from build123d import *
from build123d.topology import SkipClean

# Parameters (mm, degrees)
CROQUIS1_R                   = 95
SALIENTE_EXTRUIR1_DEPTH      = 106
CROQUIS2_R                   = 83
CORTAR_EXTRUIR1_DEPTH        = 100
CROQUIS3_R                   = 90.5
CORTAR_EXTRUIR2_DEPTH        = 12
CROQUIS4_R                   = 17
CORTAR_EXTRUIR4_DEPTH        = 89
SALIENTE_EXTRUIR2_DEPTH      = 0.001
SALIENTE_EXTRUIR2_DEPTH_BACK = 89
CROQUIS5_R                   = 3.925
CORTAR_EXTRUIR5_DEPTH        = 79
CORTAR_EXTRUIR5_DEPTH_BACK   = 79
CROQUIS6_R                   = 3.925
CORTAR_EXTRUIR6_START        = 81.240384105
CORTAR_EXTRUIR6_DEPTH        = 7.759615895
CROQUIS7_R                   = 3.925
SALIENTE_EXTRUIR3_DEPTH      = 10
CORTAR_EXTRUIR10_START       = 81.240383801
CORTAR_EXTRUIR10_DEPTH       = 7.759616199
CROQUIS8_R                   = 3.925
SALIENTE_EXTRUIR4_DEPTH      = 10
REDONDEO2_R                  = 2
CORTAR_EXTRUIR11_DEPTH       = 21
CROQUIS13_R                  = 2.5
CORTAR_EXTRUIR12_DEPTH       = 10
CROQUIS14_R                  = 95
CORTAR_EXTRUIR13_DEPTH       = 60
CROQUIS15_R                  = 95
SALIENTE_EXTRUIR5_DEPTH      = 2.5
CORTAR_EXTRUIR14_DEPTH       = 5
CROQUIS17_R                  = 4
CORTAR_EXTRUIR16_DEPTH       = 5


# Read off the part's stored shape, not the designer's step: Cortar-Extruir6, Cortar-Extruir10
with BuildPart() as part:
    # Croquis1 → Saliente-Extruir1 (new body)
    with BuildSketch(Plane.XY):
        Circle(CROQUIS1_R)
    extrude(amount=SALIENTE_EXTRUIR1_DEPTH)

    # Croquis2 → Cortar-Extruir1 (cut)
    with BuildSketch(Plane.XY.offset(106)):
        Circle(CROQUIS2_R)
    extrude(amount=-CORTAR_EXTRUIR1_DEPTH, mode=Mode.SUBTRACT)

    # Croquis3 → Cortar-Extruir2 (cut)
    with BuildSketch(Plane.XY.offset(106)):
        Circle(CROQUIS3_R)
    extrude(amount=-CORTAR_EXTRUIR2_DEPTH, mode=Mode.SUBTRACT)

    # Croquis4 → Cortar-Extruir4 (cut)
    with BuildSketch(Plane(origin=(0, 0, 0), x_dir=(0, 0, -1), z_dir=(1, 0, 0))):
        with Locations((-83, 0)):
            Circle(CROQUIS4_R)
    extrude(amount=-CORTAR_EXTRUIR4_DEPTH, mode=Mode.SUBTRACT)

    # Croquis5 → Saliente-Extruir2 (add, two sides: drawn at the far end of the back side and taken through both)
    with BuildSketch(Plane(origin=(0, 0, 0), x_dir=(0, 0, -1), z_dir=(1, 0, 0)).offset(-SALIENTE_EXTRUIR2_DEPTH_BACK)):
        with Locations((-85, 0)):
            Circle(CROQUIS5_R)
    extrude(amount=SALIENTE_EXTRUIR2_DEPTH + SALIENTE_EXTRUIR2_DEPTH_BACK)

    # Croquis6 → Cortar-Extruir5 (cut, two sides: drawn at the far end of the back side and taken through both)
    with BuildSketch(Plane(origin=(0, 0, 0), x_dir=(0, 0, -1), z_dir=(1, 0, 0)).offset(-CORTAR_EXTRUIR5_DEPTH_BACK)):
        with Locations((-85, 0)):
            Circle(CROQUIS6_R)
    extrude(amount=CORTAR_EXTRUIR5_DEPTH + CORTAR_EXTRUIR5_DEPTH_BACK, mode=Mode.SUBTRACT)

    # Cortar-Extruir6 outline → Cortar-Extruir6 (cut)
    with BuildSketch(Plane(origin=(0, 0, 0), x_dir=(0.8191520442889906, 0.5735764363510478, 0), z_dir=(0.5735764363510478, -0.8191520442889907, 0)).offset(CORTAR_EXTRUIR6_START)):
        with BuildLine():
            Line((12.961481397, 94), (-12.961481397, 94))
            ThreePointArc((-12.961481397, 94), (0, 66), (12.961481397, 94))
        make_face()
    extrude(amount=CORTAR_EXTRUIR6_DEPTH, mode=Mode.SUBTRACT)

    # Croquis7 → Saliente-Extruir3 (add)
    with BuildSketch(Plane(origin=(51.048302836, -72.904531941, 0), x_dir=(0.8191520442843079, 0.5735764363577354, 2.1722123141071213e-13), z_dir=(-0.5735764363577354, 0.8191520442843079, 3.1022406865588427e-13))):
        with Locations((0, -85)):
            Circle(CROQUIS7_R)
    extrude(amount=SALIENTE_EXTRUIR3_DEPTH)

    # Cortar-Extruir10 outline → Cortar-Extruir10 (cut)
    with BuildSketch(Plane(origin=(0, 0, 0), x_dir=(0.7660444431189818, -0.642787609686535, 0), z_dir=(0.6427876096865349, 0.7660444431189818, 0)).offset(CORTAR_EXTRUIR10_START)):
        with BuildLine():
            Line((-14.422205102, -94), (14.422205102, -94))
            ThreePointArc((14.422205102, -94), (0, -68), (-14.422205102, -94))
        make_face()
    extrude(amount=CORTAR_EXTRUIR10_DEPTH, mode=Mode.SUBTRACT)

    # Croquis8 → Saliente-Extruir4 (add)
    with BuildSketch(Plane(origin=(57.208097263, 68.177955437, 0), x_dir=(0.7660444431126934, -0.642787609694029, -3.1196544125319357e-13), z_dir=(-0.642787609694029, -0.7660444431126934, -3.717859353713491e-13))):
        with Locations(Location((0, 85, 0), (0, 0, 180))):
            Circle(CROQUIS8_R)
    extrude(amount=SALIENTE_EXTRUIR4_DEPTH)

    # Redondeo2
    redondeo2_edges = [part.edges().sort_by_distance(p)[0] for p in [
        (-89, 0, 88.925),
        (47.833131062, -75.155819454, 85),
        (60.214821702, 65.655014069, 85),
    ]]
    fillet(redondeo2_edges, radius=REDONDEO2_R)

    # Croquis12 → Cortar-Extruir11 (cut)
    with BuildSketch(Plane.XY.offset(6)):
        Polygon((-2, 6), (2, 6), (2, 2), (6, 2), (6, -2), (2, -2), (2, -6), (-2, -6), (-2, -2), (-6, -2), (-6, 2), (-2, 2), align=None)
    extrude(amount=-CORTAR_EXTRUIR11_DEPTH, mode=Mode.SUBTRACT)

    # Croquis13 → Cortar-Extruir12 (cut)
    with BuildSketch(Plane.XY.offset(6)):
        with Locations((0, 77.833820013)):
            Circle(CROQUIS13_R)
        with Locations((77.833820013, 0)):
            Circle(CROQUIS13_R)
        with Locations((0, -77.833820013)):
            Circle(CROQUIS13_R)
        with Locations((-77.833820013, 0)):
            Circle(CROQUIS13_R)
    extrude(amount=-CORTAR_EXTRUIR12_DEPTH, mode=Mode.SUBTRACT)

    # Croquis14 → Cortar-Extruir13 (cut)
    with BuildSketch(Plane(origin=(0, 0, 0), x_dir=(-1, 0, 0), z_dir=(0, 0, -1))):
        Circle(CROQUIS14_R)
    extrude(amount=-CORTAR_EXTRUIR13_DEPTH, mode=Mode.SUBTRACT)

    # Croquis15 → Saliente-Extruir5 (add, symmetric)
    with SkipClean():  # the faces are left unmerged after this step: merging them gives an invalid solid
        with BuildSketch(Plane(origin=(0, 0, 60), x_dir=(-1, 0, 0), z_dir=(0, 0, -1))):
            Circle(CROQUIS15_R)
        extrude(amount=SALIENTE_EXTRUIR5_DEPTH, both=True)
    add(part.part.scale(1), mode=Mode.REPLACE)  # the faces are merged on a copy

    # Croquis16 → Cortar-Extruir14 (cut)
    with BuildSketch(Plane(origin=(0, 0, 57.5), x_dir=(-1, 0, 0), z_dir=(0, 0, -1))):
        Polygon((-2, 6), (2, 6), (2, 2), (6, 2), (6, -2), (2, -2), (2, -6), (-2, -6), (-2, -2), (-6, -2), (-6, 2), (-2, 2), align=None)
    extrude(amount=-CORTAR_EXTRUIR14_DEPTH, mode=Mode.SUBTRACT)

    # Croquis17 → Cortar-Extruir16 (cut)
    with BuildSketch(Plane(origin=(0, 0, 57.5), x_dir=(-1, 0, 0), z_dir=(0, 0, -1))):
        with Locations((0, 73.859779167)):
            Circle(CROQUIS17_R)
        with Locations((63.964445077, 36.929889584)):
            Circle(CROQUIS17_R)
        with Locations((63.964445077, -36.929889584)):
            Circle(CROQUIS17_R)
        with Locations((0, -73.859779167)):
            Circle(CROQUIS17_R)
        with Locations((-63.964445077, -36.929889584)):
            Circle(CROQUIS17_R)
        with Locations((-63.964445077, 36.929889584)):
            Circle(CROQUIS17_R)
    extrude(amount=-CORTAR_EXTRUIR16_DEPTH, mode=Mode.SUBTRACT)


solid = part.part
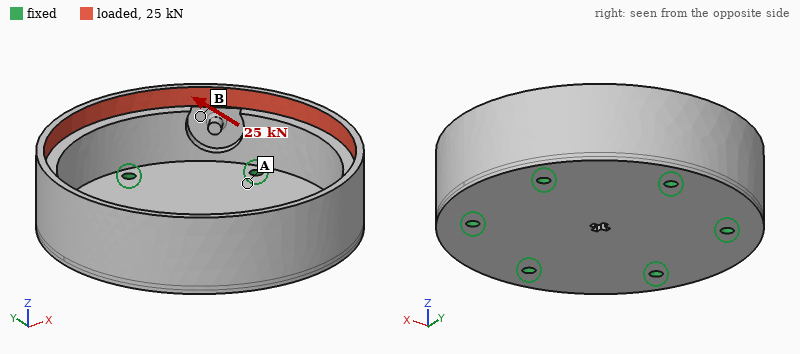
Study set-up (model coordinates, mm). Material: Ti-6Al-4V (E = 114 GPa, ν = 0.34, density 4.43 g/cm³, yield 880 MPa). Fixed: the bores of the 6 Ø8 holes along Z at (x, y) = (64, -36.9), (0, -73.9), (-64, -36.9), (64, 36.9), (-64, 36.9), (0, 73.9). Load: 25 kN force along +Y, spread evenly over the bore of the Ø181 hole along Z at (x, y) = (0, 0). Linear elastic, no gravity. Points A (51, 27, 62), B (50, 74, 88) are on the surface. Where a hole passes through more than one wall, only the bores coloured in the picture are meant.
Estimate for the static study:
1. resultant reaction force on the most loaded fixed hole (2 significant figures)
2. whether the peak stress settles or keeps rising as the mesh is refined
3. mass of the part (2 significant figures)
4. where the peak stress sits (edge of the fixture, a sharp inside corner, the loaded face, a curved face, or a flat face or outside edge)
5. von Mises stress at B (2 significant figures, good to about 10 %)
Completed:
7.9 kN
keeps rising
1.6 kg
edge of the fixture
29 MPa
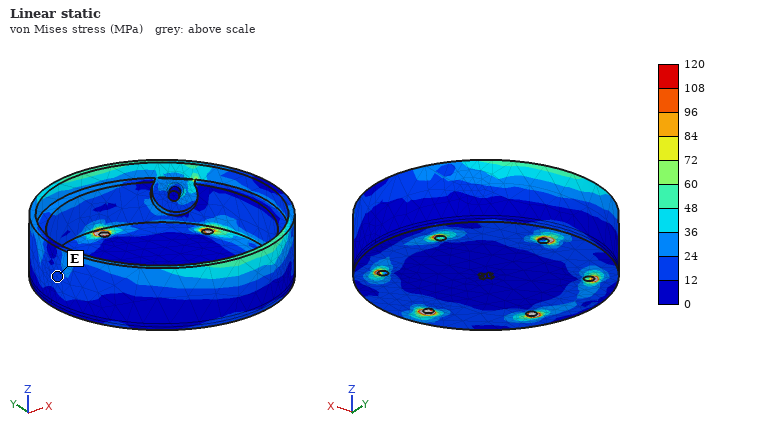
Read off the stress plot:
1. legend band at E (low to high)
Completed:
12 to 24 MPa
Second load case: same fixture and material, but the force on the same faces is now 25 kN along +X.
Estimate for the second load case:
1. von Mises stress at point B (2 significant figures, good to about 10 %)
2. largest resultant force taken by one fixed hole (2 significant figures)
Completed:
43 MPa
8.6 kN
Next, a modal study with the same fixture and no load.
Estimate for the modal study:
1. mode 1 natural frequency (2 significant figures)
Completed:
2100 Hz
